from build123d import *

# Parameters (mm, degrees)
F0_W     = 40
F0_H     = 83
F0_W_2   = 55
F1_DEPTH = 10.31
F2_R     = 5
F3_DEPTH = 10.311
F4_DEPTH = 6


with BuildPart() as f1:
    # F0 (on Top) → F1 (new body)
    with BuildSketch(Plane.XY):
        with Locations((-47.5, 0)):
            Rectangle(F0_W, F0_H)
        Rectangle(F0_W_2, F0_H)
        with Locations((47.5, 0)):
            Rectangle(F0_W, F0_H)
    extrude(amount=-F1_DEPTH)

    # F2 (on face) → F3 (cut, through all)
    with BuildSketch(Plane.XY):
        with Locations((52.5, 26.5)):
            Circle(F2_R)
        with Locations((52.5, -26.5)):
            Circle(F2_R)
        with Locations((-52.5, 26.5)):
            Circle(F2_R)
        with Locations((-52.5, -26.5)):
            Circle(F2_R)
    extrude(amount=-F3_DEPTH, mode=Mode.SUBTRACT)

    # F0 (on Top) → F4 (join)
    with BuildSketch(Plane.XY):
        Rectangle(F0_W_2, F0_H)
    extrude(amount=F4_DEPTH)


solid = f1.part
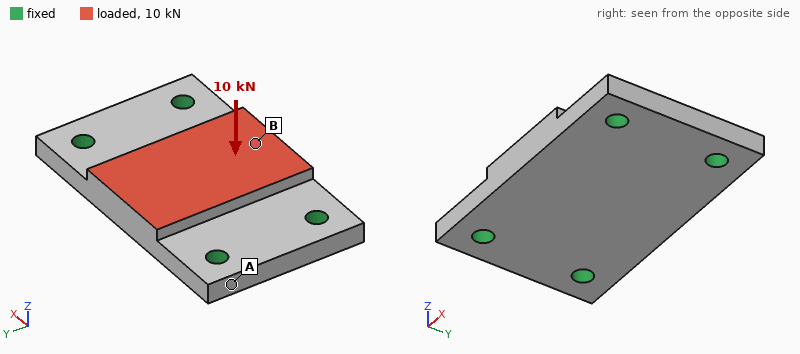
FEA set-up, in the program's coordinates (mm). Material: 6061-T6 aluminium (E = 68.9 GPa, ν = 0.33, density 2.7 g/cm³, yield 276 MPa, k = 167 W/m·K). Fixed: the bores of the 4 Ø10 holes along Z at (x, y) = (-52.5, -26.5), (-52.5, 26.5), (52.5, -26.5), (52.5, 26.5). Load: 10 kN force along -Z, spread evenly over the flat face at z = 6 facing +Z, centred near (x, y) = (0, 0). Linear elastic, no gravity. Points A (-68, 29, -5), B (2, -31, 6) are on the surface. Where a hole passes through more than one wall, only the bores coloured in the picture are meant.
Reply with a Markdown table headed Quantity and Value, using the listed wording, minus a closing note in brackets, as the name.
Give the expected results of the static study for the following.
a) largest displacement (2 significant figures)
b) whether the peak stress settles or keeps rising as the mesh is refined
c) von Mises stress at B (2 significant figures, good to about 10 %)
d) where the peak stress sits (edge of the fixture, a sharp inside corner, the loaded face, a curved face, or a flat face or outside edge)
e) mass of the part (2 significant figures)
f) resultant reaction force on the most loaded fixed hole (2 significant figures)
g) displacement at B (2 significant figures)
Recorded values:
| Quantity | Value |
|---|---|
| largest displacement | 54 µm |
| whether the peak stress settles or keeps rising as the mesh is refined | keeps rising |
| von Mises stress at B | 28 MPa |
| where the peak stress sits | edge of the fixture |
| mass of the part | 380 g |
| resultant reaction force on the most loaded fixed hole | 3.0 kN |
| displacement at B | 50 µm |
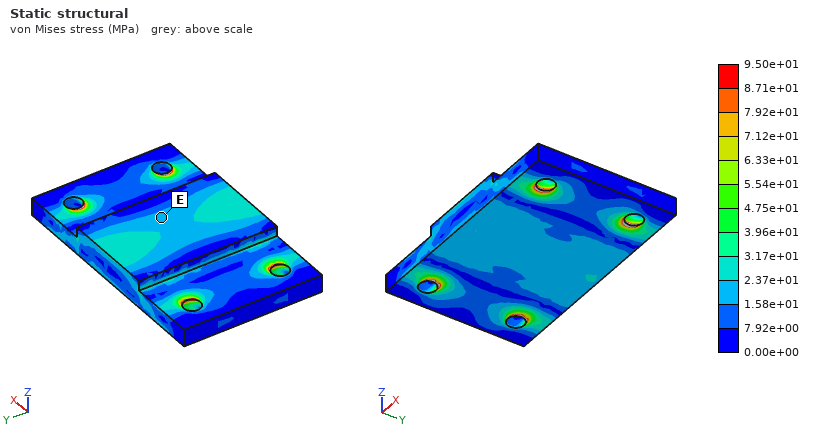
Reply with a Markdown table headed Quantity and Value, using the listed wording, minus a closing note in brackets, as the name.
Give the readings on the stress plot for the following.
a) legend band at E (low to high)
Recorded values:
| Quantity | Value |
|---|---|
| legend band at E | 1.58e+01 to 2.37e+01 MPa |
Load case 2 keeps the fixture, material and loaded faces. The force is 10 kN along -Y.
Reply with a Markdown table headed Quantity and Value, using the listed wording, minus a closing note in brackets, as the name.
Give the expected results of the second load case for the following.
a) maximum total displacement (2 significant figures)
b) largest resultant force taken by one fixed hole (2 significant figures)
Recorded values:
| Quantity | Value |
|---|---|
| maximum total displacement | 34 µm |
| largest resultant force taken by one fixed hole | 3.3 kN |
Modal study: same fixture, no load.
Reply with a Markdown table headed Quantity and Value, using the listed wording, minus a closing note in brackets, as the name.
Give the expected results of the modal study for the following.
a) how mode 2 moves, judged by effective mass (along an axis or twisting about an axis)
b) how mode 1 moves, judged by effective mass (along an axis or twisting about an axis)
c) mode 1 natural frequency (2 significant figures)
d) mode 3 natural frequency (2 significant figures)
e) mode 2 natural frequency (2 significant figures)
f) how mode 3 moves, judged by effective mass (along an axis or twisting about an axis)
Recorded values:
| Quantity | Value |
|---|---|
| how mode 2 moves, judged by effective mass | twisting about X |
| how mode 1 moves, judged by effective mass | along Z |
| mode 1 natural frequency | 5000 Hz |
| mode 3 natural frequency | 11 kHz |
| mode 2 natural frequency | 6100 Hz |
| how mode 3 moves, judged by effective mass | along Y |
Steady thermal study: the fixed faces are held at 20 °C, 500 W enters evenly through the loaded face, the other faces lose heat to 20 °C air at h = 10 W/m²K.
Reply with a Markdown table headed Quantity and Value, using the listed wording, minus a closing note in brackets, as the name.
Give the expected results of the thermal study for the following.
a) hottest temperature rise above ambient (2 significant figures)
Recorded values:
| Quantity | Value |
|---|---|
| hottest temperature rise above ambient | 68 K |
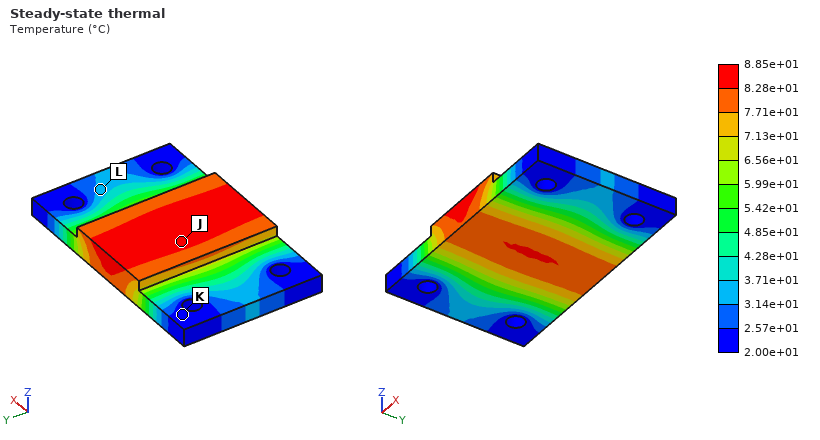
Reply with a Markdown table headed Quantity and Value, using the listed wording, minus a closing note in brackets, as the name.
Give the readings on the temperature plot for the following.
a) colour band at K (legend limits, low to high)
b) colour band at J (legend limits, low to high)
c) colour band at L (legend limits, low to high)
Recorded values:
| Quantity | Value |
|---|---|
| colour band at K | 2.00e+01 to 2.57e+01 °C |
| colour band at J | 8.28e+01 to 8.85e+01 °C |
| colour band at L | 3.14e+01 to 3.71e+01 °C |
